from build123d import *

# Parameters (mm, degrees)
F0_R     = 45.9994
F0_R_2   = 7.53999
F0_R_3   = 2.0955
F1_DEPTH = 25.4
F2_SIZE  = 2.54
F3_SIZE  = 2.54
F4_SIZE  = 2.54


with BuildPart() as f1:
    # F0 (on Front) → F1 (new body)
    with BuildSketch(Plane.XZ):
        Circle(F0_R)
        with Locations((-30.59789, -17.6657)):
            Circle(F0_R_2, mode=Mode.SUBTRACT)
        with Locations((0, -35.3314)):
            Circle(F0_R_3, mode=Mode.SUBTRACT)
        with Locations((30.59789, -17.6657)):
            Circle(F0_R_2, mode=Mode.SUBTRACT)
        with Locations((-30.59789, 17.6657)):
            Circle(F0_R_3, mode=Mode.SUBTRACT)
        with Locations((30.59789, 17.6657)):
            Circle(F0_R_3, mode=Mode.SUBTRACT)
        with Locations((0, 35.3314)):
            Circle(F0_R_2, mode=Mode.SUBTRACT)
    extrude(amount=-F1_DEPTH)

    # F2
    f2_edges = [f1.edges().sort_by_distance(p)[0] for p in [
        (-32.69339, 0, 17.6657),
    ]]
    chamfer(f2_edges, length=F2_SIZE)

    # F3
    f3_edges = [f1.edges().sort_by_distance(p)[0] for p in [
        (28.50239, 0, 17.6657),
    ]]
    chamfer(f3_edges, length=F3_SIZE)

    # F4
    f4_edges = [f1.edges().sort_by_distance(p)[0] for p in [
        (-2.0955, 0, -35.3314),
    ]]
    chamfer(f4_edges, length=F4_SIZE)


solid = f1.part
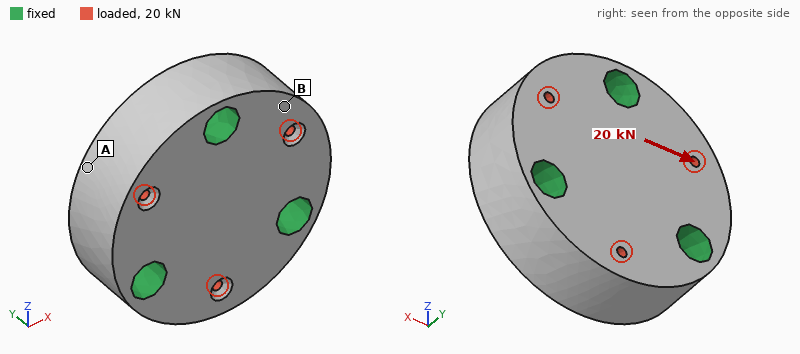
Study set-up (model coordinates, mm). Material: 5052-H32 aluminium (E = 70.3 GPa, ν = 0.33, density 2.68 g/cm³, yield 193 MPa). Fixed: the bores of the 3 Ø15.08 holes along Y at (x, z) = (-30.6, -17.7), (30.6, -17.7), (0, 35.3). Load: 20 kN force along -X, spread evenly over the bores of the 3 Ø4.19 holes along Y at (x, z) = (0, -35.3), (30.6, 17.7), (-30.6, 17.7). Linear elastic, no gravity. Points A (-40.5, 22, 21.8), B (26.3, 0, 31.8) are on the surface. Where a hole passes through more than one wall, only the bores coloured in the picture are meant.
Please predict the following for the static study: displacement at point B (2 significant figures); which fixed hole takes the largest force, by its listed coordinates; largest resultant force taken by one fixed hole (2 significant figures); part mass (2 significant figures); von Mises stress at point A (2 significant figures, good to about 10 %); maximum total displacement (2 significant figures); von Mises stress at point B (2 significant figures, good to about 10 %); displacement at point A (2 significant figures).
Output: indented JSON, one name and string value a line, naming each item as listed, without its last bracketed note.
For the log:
{
  "displacement at point B": "1.5 µm",
  "which fixed hole takes the largest force, by its listed coordinates": "(0, 35.3)",
  "largest resultant force taken by one fixed hole": "8.2 kN",
  "part mass": "410 g",
  "von Mises stress at point A": "14 MPa",
  "maximum total displacement": "6.3 µm",
  "von Mises stress at point B": "4.7 MPa",
  "displacement at point A": "5.0 µm"
}
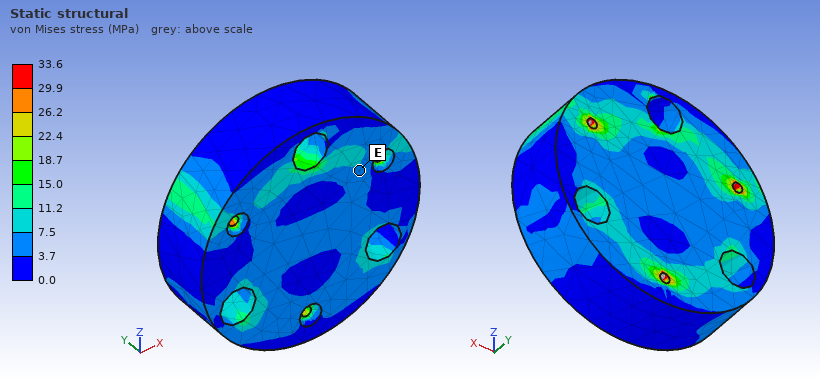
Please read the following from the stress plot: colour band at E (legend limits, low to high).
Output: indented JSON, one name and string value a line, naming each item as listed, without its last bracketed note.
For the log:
{
  "colour band at E": "3.7 to 7.5 MPa"
}
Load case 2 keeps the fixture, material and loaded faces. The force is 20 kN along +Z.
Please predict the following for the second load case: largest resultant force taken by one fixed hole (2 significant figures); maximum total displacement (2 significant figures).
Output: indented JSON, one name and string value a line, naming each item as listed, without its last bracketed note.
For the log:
{
  "largest resultant force taken by one fixed hole": "7.6 kN",
  "maximum total displacement": "6.6 µm"
}
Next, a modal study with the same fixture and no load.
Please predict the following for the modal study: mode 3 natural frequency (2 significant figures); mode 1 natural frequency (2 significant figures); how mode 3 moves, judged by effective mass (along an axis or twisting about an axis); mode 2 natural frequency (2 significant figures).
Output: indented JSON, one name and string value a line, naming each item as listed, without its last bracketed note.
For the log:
{
  "mode 3 natural frequency": "19 kHz",
  "mode 1 natural frequency": "18 kHz",
  "how mode 3 moves, judged by effective mass": "along Y",
  "mode 2 natural frequency": "18 kHz"
}
